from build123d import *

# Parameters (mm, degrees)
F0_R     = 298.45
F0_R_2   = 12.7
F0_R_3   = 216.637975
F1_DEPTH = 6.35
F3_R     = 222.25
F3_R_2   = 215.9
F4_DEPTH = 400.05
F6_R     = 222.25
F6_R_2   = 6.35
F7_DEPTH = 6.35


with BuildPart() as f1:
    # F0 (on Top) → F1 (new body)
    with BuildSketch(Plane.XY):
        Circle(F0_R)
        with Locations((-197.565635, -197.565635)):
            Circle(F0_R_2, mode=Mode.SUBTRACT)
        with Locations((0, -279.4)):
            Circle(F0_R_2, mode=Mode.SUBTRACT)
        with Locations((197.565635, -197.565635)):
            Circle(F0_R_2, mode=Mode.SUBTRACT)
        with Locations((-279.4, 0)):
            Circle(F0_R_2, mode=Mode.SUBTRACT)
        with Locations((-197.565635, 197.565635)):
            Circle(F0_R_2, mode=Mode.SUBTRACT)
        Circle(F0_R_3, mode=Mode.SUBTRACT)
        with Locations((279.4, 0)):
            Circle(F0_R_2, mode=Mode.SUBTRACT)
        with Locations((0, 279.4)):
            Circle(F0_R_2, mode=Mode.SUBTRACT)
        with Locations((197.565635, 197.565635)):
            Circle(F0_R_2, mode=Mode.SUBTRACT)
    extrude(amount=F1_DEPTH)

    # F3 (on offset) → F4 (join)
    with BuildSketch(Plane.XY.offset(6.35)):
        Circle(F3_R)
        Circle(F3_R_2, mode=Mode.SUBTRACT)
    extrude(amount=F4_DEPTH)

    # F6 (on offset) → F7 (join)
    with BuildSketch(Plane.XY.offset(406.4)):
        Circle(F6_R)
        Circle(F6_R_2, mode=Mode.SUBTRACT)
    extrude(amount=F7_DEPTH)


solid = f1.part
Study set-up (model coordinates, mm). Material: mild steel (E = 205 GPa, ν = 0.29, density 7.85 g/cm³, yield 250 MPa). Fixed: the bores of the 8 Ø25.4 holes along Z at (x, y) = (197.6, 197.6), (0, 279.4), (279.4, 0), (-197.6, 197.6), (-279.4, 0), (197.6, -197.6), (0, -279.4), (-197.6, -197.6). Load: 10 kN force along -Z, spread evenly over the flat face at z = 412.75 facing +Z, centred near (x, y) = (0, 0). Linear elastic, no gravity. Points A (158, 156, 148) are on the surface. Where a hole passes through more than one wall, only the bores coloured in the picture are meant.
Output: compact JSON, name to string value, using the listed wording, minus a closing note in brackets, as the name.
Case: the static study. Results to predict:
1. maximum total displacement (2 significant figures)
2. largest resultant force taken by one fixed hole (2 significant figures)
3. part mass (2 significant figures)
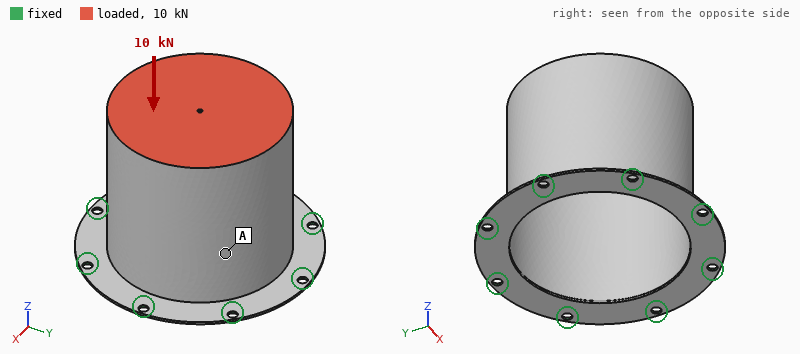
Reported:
{"maximum total displacement": "0.62 mm", "largest resultant force taken by one fixed hole": "1.6 kN", "part mass": "42 kg"}
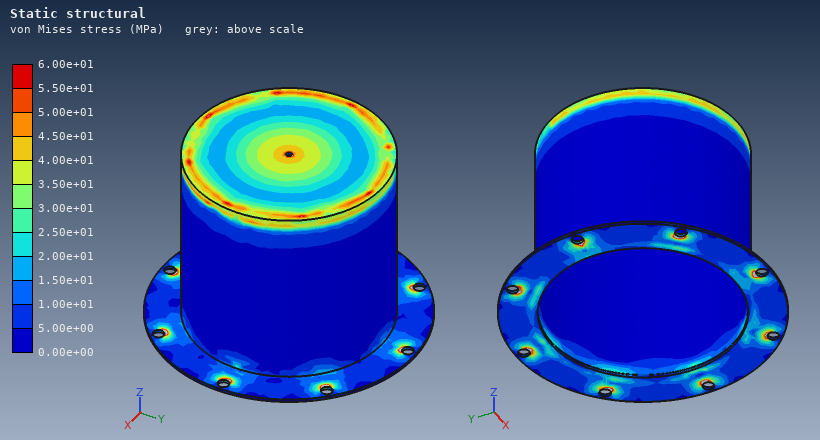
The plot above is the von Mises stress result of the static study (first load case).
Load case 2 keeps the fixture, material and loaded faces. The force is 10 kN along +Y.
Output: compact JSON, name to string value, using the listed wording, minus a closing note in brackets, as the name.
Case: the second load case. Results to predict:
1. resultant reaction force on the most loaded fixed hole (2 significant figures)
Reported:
{"resultant reaction force on the most loaded fixed hole": "5.1 kN"}
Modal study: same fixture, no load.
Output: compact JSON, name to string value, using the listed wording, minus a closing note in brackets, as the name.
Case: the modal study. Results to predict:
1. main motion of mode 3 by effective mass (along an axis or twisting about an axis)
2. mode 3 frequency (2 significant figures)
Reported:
{"main motion of mode 3 by effective mass": "along Z", "mode 3 frequency": "280 Hz"}
